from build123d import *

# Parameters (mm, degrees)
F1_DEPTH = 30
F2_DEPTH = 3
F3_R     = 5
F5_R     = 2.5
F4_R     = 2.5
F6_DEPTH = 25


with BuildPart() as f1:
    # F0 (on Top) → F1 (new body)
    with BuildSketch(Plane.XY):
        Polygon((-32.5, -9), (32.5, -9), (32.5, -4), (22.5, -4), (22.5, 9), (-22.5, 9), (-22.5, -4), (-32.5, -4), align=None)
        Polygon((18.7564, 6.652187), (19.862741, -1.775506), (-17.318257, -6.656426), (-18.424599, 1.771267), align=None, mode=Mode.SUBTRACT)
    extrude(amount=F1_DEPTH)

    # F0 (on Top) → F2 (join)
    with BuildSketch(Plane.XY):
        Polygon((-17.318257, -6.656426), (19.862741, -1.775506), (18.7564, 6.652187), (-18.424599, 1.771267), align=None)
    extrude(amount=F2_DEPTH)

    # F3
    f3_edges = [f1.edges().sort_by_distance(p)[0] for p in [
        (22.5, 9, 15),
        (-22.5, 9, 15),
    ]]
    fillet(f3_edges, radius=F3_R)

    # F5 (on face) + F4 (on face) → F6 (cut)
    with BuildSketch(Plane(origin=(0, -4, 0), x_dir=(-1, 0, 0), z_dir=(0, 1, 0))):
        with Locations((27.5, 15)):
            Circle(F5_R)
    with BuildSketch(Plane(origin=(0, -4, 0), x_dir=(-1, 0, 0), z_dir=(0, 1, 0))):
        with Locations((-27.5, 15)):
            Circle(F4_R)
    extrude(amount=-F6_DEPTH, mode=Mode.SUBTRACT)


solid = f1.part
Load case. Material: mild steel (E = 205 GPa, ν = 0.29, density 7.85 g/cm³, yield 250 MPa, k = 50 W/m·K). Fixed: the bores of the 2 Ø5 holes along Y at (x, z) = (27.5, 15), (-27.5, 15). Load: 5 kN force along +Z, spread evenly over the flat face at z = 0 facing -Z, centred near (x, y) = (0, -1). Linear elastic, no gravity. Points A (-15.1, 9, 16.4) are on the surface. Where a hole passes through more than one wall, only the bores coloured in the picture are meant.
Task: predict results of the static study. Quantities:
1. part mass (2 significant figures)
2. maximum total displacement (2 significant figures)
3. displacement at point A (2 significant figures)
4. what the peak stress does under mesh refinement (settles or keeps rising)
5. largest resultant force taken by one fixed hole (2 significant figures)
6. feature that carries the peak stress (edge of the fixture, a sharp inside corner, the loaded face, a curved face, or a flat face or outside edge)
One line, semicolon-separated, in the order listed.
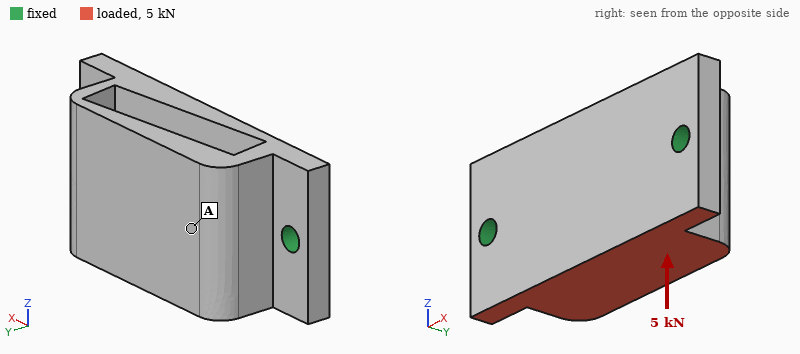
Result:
140 g; 29 µm; 21 µm; keeps rising; 2.5 kN; edge of the fixture
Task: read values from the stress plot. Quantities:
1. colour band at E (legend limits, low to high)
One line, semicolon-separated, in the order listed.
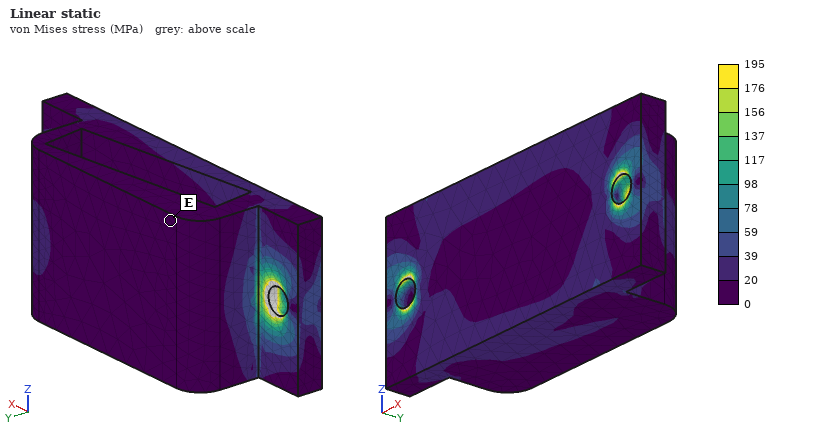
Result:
0 to 20 MPa
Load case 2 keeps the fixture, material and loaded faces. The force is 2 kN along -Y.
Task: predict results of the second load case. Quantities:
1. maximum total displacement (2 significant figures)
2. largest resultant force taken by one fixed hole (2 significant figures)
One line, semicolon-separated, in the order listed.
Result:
29 µm; 1.1 kN
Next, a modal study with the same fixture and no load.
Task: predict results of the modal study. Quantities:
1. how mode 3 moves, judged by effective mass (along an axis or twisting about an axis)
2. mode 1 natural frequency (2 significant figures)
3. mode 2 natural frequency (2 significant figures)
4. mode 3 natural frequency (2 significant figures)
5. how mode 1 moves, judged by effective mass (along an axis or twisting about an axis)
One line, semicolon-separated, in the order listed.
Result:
along Y; 5500 Hz; 8500 Hz; 9900 Hz; along Z
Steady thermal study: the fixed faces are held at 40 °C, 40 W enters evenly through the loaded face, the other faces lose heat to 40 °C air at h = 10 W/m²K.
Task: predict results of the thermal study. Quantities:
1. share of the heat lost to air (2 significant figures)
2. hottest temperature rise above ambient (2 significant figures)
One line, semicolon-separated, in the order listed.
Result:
6.3 %; 57 K
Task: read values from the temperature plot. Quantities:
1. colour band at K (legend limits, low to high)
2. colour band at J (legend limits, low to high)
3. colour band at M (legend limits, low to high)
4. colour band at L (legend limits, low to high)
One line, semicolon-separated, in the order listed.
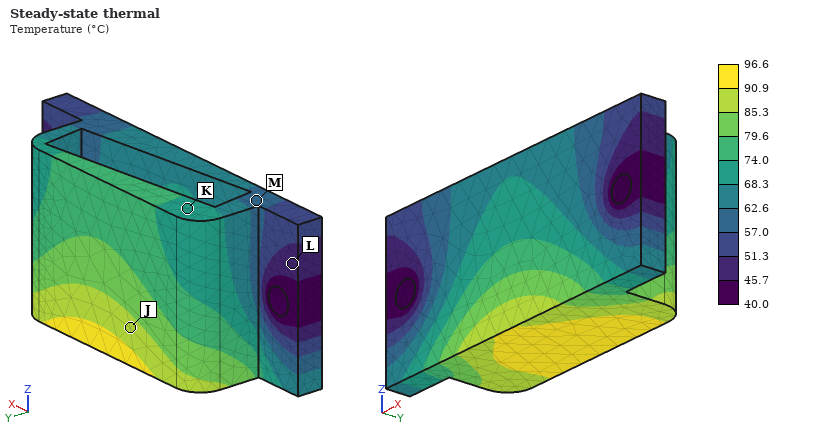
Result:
68.3 to 74.0 °C; 85.3 to 90.9 °C; 57.0 to 62.6 °C; 45.7 to 51.3 °C
